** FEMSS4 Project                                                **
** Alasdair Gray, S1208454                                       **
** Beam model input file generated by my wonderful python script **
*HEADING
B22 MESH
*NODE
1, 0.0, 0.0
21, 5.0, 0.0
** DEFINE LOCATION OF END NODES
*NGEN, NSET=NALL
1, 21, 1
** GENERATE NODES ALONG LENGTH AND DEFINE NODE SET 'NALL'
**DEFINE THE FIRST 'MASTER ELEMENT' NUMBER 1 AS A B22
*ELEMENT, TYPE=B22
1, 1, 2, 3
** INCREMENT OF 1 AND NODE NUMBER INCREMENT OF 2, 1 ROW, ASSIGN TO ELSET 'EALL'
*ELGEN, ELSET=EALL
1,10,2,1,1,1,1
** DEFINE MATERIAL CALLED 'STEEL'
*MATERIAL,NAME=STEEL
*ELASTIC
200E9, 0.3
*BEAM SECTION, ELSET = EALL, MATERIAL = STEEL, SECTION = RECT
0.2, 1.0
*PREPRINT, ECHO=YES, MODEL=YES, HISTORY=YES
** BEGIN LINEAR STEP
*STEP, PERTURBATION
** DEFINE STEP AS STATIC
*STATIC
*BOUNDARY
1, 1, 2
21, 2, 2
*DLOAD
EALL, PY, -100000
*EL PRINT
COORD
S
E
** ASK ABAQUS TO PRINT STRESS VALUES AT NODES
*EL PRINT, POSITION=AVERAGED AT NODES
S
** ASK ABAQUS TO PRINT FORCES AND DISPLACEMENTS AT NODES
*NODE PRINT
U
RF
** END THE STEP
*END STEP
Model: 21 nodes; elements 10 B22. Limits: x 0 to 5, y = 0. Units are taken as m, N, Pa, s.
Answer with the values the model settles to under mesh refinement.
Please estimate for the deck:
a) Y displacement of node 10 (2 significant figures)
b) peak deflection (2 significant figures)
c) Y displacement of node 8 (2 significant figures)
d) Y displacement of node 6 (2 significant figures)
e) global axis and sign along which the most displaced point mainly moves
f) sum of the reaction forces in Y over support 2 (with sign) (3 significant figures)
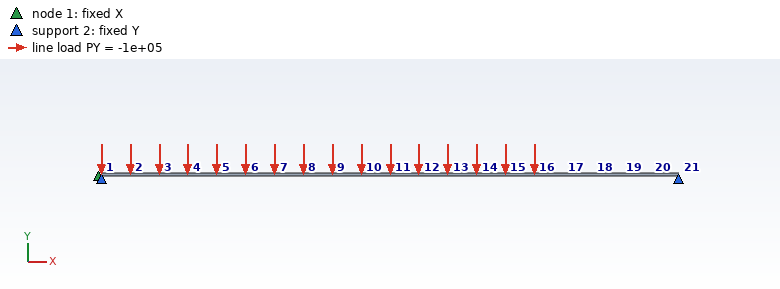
-2.7e-04 m
2.7e-04 m
-2.4e-04 m
-1.9e-04 m
-Y
5.00e+05 N
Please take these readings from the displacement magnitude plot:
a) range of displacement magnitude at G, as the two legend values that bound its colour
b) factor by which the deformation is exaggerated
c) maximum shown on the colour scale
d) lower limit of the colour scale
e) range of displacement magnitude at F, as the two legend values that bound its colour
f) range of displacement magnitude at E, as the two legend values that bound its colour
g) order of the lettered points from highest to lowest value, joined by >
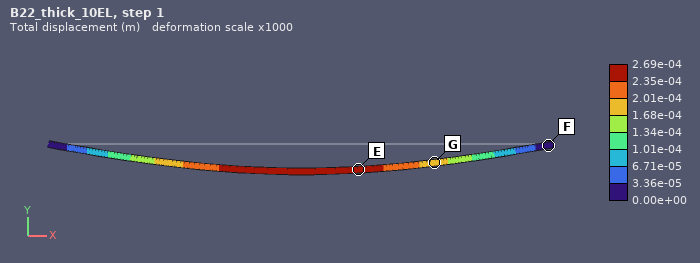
1.68e-04 to 2.01e-04 m
1000
2.69e-04 m
0.00e+00 m
0.00e+00 to 3.36e-05 m
2.35e-04 to 2.69e-04 m
E > G > F
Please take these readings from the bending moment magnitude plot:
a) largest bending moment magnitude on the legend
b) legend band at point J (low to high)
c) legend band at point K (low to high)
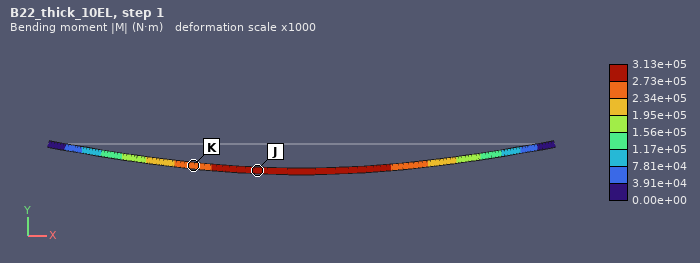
3.13e+05 N·m
2.73e+05 to 3.13e+05 N·m
2.34e+05 to 2.73e+05 N·m
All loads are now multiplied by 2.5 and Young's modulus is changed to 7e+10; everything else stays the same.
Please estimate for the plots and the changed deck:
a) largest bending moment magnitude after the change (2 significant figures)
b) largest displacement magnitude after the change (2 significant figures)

7.8e+05 N·m
0.0019 m
